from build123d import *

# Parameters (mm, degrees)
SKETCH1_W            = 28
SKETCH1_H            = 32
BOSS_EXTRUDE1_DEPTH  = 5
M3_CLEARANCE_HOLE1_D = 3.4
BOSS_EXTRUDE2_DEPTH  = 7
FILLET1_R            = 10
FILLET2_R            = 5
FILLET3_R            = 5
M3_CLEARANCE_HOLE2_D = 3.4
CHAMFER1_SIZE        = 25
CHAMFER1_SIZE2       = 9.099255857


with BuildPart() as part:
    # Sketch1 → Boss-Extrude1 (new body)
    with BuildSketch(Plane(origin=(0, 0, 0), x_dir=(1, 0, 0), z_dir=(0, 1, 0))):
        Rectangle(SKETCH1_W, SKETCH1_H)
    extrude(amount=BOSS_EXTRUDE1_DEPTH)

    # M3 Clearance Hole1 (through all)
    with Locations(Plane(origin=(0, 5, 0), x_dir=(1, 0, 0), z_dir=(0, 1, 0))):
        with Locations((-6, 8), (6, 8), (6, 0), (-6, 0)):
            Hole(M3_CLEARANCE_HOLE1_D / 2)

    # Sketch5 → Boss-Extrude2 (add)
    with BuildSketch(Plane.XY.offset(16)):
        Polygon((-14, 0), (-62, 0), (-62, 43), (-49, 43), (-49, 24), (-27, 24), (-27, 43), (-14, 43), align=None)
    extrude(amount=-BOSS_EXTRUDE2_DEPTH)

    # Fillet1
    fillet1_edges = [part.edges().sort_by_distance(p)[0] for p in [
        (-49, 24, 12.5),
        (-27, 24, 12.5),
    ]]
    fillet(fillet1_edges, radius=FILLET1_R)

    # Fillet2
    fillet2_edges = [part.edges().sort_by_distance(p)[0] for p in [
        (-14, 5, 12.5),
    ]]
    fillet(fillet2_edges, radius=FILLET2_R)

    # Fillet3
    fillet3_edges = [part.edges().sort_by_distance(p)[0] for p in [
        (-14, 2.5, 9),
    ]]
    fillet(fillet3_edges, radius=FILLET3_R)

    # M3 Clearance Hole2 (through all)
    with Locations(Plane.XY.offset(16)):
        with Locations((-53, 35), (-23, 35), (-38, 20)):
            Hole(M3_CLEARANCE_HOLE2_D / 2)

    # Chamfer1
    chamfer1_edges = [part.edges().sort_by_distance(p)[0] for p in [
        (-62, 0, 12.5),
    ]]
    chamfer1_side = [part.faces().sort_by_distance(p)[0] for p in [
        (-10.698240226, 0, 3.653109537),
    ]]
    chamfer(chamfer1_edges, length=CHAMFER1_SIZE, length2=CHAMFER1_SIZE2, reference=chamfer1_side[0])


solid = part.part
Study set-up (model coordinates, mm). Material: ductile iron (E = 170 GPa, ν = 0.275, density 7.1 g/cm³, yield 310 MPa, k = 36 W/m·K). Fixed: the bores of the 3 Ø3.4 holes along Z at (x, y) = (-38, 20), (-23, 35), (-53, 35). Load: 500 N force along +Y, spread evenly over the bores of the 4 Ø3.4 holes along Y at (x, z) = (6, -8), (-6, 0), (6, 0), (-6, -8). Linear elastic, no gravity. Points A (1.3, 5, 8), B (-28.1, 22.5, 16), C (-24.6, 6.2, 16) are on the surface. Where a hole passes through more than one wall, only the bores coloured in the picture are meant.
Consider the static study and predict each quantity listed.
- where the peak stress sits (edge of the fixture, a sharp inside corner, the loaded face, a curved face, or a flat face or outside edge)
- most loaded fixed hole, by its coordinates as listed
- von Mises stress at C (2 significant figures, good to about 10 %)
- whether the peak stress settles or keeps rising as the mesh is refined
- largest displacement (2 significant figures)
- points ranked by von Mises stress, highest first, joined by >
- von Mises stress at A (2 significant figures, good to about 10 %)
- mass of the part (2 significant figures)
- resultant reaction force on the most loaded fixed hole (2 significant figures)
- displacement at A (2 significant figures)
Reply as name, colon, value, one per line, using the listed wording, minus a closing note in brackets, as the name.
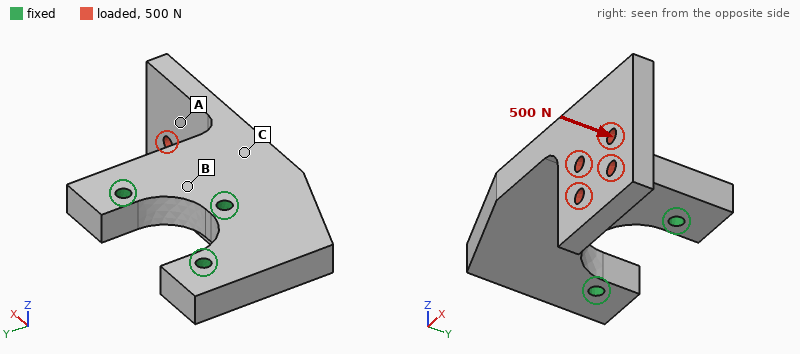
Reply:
where the peak stress sits: a sharp inside corner
most loaded fixed hole, by its coordinates as listed: (-23, 35)
von Mises stress at C: 55 MPa
whether the peak stress settles or keeps rising as the mesh is refined: keeps rising
largest displacement: 0.24 mm
points ranked by von Mises stress, highest first, joined by >: C > A > B
von Mises stress at A: 38 MPa
mass of the part: 110 g
resultant reaction force on the most loaded fixed hole: 800 N
displacement at A: 0.061 mm
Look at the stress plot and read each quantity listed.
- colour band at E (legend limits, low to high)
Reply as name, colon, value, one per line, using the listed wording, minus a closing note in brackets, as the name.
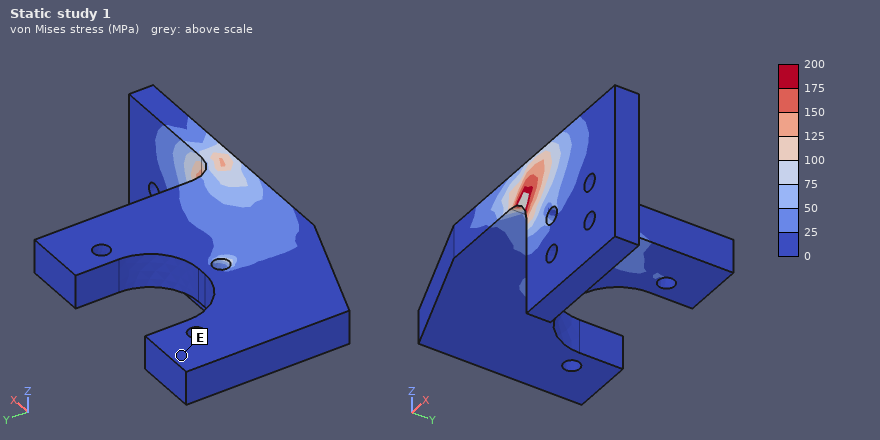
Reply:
colour band at E: 0 to 25 MPa
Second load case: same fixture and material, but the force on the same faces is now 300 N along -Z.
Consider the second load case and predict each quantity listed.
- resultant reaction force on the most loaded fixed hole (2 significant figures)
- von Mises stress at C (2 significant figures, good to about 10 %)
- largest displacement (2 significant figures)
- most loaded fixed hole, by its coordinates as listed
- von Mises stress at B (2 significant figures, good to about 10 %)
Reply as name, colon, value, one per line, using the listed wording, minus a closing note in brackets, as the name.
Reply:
resultant reaction force on the most loaded fixed hole: 230 N
von Mises stress at C: 43 MPa
largest displacement: 0.12 mm
most loaded fixed hole, by its coordinates as listed: (-38, 20)
von Mises stress at B: 20 MPa
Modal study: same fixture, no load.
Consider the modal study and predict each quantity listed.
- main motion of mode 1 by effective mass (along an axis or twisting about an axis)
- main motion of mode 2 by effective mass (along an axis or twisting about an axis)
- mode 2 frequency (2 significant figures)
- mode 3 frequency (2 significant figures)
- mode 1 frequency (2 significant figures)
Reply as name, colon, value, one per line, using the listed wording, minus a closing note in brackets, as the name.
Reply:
main motion of mode 1 by effective mass: along Z
main motion of mode 2 by effective mass: along Y
mode 2 frequency: 2000 Hz
mode 3 frequency: 4200 Hz
mode 1 frequency: 1600 Hz
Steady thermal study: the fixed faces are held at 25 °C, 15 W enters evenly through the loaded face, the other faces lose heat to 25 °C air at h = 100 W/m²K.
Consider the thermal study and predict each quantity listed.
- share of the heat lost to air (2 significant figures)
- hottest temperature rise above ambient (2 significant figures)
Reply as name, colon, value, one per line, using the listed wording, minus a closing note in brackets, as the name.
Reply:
share of the heat lost to air: 81 %
hottest temperature rise above ambient: 60 K
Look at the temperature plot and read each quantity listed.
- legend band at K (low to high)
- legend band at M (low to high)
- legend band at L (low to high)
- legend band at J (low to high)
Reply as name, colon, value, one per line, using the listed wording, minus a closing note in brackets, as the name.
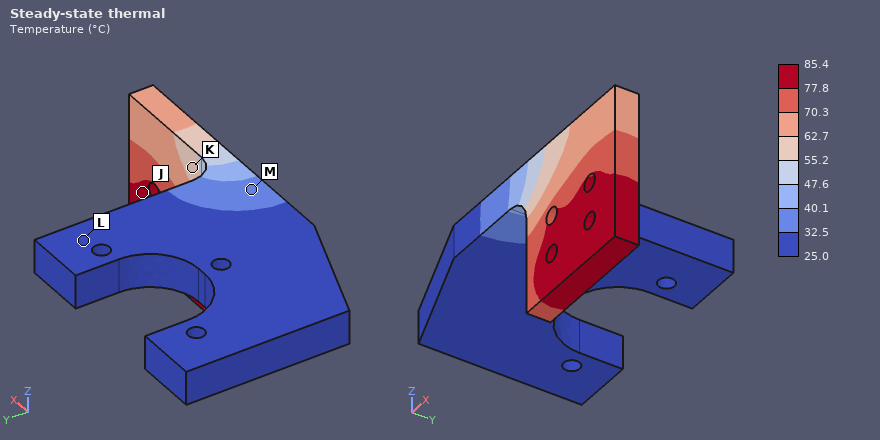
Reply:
legend band at K: 55.2 to 62.7 °C
legend band at M: 32.5 to 40.1 °C
legend band at L: 25.0 to 32.5 °C
legend band at J: 77.8 to 85.4 °C
